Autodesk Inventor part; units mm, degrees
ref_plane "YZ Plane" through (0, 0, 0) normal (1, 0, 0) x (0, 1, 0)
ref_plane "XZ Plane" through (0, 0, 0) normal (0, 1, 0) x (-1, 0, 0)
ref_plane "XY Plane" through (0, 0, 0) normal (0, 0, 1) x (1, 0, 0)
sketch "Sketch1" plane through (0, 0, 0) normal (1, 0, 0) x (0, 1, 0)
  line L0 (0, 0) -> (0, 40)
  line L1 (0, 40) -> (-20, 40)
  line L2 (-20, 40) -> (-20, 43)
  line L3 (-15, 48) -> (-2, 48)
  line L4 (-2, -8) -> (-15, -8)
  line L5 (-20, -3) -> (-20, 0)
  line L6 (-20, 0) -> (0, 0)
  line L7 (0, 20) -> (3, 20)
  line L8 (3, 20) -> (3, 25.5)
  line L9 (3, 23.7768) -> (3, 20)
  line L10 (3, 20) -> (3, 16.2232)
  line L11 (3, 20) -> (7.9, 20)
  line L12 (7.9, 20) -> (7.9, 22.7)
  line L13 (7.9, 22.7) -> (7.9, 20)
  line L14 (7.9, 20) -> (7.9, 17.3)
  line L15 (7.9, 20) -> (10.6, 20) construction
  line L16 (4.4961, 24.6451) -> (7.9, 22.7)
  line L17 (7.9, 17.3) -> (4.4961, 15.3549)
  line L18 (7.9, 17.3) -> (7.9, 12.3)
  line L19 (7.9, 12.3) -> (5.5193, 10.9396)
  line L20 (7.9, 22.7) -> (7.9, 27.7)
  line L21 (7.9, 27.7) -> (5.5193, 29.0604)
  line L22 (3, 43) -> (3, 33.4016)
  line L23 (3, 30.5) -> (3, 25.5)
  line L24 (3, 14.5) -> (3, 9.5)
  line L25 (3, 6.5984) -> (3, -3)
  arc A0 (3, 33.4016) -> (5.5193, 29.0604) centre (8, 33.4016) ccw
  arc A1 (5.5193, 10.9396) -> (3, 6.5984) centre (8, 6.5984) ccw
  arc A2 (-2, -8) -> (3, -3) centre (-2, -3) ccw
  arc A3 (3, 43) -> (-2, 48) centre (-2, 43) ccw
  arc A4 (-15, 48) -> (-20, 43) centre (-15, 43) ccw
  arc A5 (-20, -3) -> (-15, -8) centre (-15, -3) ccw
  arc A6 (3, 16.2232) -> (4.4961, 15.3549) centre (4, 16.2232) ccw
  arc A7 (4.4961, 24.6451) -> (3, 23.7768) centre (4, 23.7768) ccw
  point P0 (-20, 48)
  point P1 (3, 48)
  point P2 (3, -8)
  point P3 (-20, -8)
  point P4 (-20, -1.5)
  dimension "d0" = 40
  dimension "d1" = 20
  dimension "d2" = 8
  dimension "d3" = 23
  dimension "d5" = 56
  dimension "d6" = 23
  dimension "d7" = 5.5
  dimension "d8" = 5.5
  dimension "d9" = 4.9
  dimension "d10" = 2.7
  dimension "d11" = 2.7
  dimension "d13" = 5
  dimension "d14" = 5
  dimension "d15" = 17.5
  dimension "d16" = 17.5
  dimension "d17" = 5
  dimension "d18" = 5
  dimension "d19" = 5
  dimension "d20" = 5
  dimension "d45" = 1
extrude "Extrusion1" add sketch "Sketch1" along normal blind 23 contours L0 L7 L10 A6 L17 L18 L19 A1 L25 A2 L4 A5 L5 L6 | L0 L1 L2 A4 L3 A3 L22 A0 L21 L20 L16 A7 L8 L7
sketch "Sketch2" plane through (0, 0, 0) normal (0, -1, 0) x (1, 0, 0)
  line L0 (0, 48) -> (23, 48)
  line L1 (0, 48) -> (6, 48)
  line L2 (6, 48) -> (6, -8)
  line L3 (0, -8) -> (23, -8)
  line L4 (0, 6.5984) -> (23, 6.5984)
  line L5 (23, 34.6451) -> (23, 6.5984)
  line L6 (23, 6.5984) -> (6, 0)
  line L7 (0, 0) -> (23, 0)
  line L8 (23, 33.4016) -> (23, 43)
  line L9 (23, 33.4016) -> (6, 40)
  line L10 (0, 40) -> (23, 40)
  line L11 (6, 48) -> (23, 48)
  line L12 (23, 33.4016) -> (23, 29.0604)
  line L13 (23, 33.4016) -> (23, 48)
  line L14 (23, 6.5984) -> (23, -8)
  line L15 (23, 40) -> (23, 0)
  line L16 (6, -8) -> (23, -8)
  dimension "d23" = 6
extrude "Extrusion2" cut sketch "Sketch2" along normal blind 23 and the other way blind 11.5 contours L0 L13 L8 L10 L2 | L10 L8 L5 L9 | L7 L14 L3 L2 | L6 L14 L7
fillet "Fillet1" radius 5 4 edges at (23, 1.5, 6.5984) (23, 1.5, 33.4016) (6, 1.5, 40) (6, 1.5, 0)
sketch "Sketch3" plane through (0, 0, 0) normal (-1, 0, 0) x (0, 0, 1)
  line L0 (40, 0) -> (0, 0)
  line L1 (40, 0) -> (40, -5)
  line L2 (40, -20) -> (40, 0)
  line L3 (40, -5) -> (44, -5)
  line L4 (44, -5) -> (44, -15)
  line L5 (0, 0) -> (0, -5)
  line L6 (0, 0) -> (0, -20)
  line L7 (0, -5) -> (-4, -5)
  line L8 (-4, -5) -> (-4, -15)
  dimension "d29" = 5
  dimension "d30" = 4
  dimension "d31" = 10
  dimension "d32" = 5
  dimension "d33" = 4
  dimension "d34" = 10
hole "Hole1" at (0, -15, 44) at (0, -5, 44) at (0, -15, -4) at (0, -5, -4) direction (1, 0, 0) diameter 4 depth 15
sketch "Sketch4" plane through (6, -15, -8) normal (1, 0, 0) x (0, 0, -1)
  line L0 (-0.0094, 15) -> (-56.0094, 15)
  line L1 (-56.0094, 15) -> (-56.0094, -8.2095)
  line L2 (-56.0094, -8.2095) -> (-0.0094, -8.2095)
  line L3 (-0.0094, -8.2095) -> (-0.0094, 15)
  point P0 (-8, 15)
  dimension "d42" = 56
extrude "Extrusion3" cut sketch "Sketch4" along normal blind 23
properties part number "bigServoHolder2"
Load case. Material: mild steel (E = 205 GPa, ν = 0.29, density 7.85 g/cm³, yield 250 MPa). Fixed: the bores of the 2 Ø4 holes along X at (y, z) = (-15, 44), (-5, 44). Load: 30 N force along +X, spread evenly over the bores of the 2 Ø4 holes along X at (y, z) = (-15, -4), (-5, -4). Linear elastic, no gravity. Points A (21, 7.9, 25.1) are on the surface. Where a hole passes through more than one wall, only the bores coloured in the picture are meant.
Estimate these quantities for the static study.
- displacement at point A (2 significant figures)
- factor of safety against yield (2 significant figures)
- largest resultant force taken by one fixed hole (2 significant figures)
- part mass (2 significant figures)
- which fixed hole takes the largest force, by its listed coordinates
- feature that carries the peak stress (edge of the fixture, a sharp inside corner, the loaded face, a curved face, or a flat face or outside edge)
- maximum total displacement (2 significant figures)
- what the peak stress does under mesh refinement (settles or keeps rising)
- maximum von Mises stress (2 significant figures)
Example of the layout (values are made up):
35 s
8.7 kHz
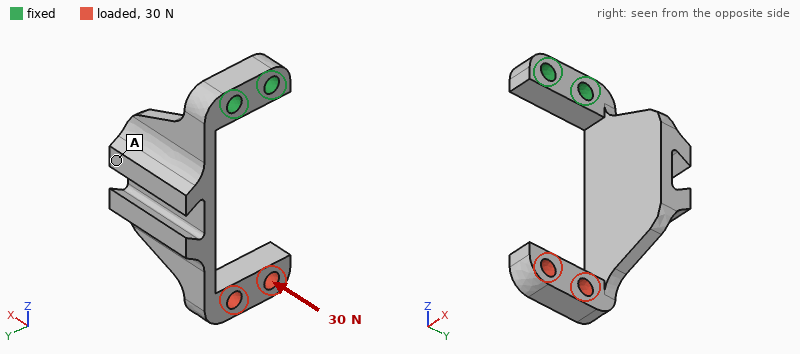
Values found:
23 µm
2.7
28 N
43 g
(-5, 44)
a curved face
75 µm
settles
91 MPa
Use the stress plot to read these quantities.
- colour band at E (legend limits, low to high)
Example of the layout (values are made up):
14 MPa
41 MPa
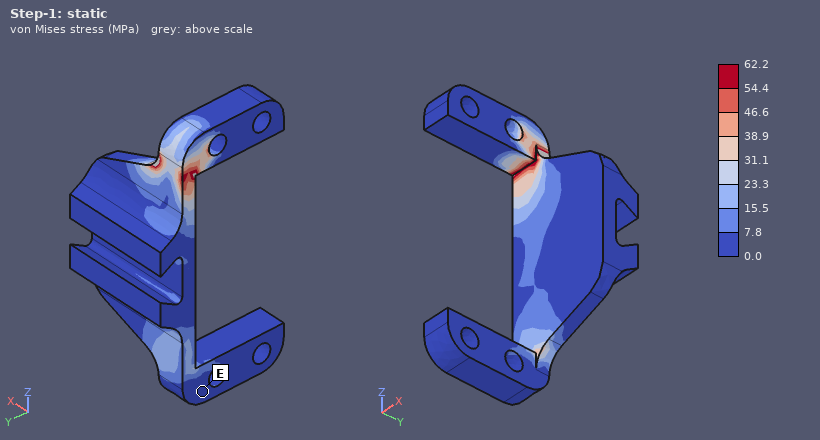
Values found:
0.0 to 7.8 MPa
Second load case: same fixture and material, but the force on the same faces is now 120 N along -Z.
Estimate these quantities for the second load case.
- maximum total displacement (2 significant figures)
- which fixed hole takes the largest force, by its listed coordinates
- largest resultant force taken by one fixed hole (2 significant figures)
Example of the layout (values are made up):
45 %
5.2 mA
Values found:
0.30 mm
(-5, 44)
110 N
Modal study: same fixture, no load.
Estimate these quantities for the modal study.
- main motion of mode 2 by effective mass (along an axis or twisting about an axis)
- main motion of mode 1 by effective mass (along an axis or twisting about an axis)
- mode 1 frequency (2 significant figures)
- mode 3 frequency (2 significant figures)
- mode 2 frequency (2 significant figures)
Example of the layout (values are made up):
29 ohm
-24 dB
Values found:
along X
along Y
580 Hz
1900 Hz
1100 Hz
